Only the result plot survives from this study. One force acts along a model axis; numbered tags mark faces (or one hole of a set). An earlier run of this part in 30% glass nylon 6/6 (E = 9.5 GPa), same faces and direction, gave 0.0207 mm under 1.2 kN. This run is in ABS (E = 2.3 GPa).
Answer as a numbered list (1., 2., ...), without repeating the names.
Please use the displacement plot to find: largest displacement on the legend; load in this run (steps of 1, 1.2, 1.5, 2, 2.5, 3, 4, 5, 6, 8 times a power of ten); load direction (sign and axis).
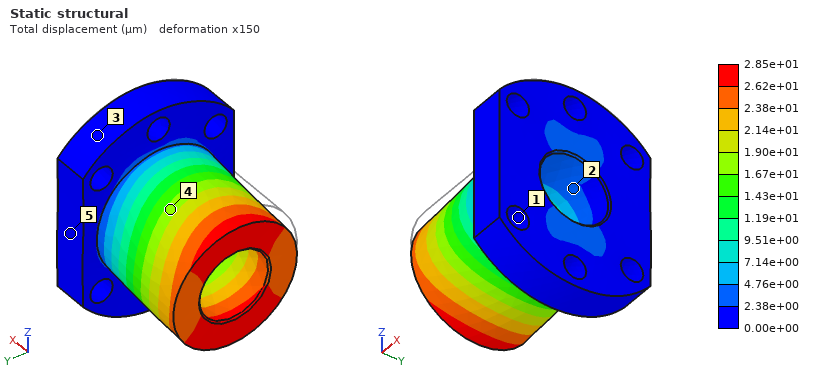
1. 2.85e+01 µm
2. 400 N
3. -Z
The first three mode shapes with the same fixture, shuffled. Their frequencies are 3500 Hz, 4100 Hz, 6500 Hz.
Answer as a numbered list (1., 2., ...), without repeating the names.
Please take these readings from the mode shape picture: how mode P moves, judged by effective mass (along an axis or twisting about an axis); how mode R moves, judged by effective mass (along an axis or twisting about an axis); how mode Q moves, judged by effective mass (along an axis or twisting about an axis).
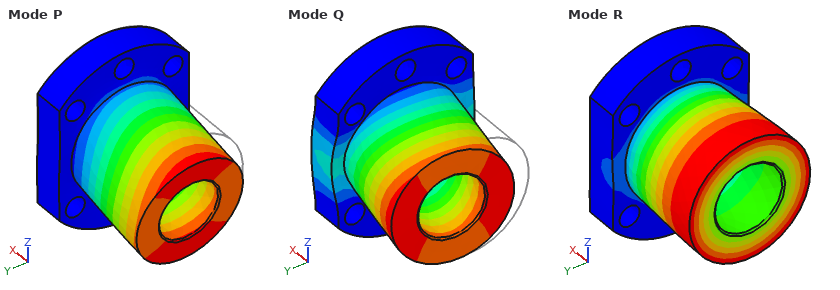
1. along Z
2. twisting about X
3. along Y
